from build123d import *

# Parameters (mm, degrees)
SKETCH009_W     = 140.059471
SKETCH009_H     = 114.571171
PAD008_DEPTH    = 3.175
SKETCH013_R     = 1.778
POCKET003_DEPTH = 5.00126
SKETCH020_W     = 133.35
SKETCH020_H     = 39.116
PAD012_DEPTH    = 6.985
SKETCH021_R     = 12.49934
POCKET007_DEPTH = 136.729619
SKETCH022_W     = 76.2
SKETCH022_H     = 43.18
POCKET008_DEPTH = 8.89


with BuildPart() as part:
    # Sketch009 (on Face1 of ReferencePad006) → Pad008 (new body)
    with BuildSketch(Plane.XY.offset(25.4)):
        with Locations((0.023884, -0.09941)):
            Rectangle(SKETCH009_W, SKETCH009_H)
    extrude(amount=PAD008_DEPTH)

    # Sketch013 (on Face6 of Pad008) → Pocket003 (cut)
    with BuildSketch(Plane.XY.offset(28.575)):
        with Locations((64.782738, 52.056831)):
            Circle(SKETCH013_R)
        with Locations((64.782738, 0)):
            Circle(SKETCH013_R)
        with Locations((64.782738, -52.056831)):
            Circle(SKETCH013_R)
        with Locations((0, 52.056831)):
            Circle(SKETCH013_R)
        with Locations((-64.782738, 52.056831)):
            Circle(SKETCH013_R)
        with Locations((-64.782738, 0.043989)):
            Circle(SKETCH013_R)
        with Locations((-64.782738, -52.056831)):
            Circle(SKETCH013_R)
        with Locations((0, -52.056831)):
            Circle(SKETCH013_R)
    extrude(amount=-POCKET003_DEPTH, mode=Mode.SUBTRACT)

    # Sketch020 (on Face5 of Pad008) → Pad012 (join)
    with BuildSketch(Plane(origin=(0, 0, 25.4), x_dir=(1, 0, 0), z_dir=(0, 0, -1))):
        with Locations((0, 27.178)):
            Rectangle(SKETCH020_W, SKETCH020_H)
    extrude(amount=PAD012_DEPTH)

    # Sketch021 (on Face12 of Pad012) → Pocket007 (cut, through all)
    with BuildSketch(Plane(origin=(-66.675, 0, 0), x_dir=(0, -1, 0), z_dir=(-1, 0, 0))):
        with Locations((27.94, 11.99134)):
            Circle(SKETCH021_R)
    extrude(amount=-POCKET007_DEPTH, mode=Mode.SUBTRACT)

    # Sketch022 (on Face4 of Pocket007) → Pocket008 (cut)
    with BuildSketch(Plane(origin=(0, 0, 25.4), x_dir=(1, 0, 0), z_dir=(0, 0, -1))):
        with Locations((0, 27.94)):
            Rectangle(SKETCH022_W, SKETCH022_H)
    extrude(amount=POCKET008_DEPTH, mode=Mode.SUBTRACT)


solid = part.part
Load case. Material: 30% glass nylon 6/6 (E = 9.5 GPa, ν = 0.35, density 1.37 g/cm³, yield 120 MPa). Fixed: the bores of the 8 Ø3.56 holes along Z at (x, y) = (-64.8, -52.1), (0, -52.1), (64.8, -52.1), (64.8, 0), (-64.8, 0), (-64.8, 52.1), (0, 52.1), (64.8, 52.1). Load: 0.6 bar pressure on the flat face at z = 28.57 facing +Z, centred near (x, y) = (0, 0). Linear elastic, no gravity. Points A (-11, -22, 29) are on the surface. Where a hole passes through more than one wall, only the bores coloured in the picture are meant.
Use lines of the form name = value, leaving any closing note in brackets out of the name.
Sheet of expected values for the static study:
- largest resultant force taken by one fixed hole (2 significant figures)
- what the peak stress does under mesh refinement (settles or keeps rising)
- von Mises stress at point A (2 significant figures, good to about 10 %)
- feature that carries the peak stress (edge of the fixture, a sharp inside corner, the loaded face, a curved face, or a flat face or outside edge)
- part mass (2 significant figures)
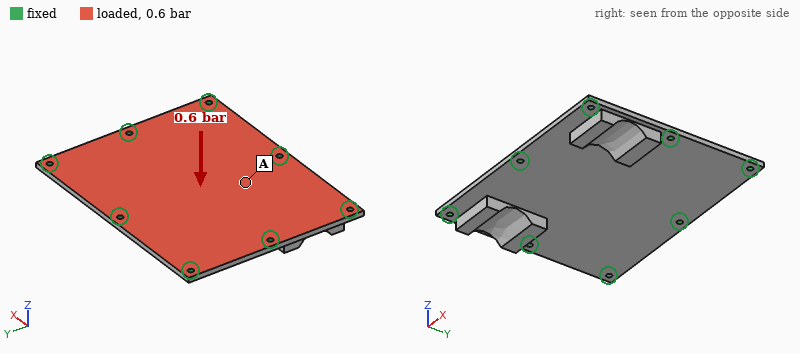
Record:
largest resultant force taken by one fixed hole = 210 N
what the peak stress does under mesh refinement = keeps rising
von Mises stress at point A = 8.8 MPa
feature that carries the peak stress = edge of the fixture
part mass = 84 g
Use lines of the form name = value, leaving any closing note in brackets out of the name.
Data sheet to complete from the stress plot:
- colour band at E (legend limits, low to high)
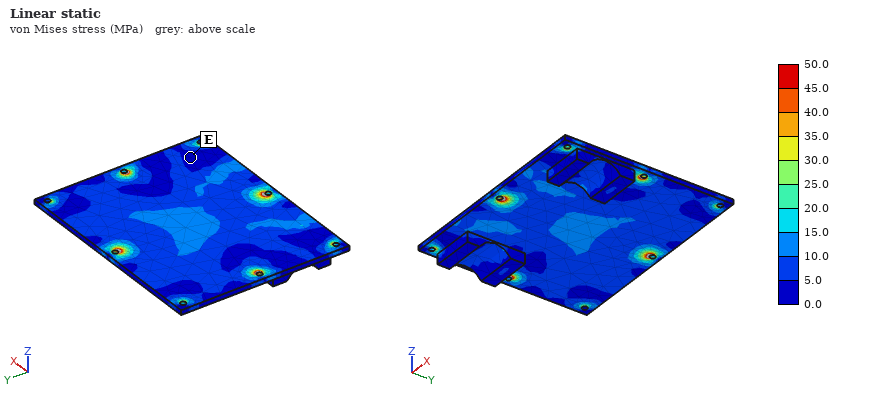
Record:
colour band at E = 0.0 to 5.0 MPa
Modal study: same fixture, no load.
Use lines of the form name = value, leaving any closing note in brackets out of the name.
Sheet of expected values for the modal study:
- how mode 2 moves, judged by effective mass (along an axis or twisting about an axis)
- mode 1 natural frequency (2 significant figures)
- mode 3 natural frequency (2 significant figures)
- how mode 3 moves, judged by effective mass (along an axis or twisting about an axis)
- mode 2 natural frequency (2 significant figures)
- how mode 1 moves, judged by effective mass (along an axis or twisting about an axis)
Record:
how mode 2 moves, judged by effective mass = twisting about Y
mode 1 natural frequency = 950 Hz
mode 3 natural frequency = 1700 Hz
how mode 3 moves, judged by effective mass = twisting about X
mode 2 natural frequency = 1400 Hz
how mode 1 moves, judged by effective mass = along Z
